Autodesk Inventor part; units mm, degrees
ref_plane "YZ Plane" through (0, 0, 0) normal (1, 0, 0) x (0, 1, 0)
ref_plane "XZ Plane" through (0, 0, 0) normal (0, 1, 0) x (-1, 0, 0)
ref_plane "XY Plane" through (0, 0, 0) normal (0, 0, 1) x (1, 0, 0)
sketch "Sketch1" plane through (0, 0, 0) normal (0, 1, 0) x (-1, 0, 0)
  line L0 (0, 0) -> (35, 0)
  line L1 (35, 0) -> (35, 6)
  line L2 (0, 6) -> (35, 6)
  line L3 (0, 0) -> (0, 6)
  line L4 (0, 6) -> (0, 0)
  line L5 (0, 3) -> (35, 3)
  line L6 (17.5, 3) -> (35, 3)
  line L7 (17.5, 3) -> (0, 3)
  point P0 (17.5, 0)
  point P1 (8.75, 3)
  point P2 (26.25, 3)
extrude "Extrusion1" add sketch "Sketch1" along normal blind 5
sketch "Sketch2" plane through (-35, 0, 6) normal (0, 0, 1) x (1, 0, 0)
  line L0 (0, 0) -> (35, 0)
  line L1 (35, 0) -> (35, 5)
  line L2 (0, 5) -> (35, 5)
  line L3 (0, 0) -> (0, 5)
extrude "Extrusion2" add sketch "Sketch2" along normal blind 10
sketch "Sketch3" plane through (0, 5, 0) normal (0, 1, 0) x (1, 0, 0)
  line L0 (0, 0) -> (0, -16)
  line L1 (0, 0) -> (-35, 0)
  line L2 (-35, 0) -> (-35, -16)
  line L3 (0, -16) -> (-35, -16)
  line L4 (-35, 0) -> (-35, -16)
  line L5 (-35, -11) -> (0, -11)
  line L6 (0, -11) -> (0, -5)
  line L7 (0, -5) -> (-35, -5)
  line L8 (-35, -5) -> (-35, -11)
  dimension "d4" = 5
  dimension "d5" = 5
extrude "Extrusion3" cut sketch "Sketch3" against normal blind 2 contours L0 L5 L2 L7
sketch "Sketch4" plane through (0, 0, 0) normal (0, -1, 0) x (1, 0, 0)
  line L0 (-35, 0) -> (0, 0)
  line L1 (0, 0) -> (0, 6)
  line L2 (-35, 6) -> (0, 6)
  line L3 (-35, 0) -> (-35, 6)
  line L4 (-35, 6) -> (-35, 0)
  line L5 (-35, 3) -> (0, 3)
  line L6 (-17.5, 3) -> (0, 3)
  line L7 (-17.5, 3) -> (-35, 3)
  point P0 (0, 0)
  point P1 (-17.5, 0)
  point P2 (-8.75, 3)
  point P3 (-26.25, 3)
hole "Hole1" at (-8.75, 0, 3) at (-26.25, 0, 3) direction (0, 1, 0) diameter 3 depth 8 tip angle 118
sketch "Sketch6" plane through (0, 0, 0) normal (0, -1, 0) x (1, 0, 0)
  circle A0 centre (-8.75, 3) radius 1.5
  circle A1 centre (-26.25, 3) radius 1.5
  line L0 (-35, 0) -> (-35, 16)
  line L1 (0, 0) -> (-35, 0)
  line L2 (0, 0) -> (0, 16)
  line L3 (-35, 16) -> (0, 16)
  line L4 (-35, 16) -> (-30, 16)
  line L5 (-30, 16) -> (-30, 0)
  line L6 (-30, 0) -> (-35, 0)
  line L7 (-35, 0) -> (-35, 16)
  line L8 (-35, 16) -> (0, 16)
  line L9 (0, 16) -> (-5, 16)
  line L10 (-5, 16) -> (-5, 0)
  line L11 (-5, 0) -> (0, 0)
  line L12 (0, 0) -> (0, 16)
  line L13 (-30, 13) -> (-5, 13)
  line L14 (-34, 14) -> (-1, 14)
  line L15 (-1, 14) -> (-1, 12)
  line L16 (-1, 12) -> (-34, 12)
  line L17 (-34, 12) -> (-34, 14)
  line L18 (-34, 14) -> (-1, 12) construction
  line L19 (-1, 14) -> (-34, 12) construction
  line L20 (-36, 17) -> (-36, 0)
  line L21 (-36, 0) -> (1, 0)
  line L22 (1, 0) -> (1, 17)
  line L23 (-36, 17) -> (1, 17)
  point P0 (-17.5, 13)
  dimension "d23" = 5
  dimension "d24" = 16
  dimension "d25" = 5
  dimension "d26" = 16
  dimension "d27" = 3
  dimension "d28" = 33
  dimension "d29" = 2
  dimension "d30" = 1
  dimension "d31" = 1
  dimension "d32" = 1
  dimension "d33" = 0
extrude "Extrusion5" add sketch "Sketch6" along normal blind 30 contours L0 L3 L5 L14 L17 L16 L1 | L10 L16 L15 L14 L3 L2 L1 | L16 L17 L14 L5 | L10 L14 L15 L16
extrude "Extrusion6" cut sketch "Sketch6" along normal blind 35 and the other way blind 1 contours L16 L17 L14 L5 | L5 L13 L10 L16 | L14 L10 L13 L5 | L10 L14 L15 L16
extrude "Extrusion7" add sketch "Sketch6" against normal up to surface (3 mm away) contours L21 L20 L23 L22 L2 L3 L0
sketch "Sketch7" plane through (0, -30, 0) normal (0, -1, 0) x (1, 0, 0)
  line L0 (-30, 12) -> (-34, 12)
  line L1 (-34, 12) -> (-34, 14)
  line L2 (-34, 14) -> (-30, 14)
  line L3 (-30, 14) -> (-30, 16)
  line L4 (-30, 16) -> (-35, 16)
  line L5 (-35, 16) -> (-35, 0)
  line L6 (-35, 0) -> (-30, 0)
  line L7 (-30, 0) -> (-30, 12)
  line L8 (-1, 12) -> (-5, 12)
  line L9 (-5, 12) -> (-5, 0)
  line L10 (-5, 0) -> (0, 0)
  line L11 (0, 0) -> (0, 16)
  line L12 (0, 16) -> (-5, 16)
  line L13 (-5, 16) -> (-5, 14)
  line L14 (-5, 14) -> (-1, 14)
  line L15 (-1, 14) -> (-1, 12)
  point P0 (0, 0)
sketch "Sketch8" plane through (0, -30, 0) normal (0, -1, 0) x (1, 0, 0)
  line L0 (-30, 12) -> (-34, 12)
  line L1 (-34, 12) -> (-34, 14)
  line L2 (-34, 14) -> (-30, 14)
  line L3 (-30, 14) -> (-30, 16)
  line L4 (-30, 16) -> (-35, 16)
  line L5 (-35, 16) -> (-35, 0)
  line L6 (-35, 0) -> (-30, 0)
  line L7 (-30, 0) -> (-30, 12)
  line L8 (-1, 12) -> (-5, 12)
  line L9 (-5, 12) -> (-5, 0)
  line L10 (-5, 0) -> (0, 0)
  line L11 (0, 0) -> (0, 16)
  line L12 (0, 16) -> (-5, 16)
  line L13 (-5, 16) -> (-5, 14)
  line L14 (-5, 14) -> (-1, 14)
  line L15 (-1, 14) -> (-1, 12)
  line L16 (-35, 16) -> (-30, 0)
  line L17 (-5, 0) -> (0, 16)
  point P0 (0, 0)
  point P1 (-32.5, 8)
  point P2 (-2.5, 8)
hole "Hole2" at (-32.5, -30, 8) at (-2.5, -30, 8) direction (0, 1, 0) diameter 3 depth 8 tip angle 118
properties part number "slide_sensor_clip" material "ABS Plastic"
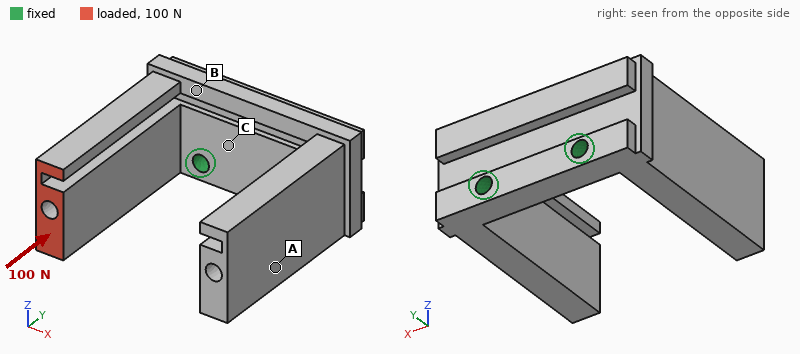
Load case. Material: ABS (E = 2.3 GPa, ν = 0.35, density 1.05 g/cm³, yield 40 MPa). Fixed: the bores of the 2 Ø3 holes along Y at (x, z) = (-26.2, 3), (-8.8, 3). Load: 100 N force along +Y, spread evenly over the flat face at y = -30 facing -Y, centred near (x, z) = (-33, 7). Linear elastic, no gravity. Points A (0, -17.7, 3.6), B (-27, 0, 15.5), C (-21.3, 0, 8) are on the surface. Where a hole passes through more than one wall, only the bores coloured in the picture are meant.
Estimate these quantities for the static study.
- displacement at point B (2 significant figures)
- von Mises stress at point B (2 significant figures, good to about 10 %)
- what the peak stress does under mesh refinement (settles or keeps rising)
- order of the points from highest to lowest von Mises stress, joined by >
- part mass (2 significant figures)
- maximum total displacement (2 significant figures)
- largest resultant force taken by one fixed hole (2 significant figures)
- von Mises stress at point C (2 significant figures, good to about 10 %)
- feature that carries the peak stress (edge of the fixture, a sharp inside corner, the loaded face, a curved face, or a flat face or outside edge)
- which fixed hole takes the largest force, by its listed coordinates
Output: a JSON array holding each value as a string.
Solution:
["0.13 mm", "2.5 MPa", "keeps rising", "C > B > A", "7.0 g", "0.55 mm", "110 N", "4.7 MPa", "edge of the fixture", "(-26.2, 3)"]
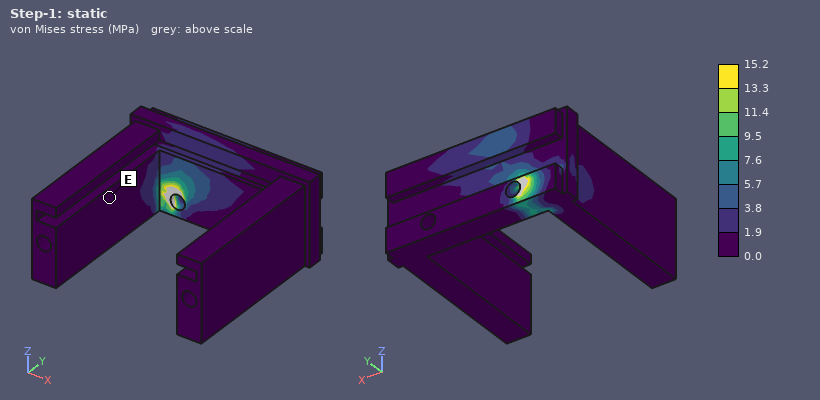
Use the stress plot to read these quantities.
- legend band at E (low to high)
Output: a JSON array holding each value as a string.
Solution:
["0.0 to 1.9 MPa"]
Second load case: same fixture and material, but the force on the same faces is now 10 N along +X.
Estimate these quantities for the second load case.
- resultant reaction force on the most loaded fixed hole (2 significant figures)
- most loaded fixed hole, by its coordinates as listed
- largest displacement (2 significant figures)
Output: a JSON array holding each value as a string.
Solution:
["9.6 N", "(-26.2, 3)", "0.55 mm"]
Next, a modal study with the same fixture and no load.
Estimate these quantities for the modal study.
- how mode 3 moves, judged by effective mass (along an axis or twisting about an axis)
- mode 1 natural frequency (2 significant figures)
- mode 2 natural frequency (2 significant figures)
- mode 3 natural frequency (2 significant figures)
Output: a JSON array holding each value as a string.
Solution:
["along Z", "820 Hz", "840 Hz", "1000 Hz"]
